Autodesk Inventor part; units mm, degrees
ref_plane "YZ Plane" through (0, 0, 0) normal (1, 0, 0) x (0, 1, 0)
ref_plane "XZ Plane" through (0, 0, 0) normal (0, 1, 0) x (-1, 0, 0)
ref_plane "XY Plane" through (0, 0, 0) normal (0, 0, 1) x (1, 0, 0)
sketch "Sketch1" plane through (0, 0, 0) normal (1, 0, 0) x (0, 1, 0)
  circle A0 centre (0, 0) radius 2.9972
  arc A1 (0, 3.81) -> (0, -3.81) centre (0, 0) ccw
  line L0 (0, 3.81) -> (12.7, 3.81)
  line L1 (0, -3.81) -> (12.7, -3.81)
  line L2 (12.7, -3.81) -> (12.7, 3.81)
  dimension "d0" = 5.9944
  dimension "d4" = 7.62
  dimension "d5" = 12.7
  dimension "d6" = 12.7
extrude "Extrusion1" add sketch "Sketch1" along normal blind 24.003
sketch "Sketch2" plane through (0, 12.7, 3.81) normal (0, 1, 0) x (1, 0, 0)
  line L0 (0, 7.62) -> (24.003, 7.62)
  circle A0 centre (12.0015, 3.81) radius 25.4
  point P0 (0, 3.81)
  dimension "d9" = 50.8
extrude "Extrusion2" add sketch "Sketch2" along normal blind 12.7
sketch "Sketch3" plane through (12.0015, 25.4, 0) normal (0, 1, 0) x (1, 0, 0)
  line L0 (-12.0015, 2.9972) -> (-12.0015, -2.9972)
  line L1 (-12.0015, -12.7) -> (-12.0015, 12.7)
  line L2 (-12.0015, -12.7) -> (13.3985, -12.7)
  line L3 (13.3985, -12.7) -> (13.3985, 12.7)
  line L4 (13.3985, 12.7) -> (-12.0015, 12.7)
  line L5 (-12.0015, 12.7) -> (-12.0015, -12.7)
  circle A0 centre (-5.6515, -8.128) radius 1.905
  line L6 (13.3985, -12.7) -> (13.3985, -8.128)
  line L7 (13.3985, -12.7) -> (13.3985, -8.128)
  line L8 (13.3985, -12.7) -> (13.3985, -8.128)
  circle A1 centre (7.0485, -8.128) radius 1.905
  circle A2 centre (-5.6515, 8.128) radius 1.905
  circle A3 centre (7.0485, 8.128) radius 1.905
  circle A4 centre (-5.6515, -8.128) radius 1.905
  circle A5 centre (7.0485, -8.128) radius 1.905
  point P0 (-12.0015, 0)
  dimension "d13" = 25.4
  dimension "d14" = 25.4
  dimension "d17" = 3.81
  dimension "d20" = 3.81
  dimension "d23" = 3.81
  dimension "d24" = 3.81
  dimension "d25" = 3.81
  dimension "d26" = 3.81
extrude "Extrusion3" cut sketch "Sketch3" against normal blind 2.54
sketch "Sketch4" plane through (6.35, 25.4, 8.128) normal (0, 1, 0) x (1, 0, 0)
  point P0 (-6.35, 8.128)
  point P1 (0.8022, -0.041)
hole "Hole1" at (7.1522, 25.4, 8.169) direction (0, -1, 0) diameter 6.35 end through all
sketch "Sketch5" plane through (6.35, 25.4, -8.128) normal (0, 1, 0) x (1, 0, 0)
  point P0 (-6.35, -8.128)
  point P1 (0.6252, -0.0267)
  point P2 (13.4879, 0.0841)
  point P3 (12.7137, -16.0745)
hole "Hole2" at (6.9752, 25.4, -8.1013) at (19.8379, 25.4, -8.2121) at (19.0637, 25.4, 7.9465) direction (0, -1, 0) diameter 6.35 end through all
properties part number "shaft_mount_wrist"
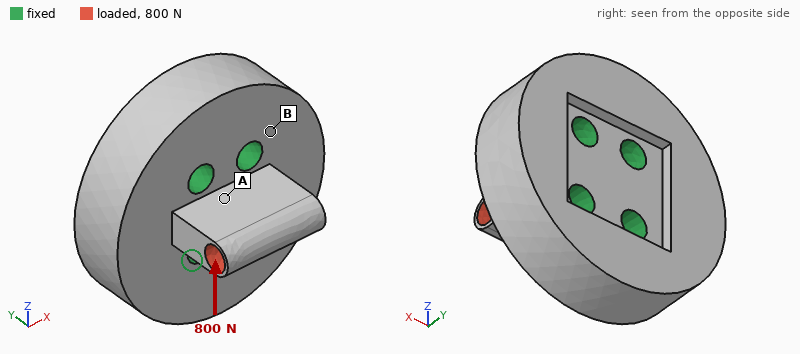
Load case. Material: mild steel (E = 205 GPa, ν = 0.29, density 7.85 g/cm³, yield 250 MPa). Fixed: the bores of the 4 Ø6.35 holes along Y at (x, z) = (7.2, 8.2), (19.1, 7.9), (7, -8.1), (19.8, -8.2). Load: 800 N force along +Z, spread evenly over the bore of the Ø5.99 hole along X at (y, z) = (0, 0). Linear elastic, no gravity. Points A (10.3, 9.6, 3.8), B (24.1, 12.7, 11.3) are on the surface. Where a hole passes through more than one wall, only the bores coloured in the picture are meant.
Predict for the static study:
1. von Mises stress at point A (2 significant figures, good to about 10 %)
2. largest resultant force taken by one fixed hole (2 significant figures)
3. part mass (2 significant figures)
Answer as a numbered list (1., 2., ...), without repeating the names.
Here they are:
1. 30 MPa
2. 590 N
3. 200 g
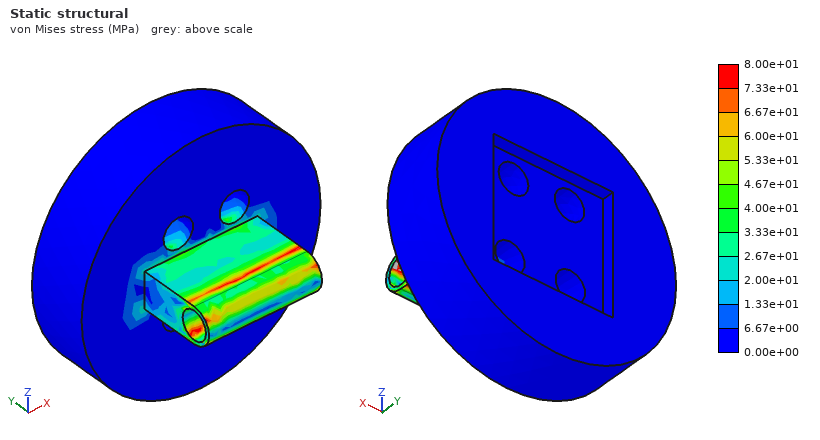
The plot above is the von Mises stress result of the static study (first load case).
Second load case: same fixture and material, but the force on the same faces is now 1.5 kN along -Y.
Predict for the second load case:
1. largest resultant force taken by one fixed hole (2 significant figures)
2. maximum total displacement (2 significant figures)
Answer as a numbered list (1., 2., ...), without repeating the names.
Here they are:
1. 450 N
2. 3.1 µm
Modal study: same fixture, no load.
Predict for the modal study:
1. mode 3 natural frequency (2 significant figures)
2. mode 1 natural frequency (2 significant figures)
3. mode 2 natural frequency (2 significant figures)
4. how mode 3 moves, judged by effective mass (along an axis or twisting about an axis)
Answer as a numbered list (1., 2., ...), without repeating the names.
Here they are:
1. 26 kHz
2. 22 kHz
3. 22 kHz
4. twisting about X
